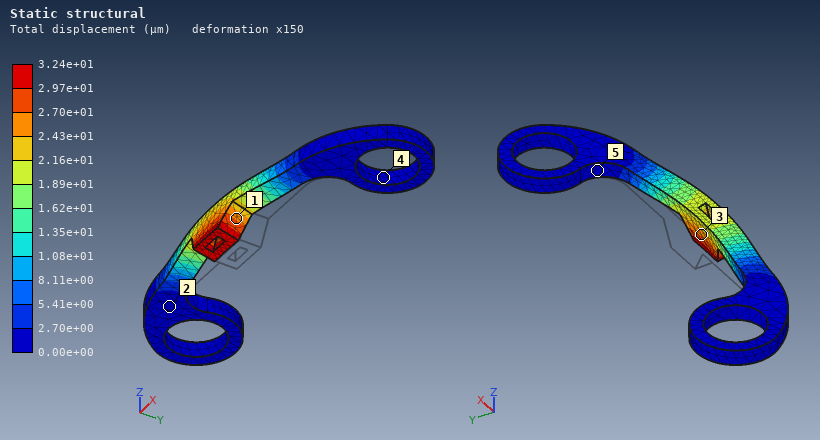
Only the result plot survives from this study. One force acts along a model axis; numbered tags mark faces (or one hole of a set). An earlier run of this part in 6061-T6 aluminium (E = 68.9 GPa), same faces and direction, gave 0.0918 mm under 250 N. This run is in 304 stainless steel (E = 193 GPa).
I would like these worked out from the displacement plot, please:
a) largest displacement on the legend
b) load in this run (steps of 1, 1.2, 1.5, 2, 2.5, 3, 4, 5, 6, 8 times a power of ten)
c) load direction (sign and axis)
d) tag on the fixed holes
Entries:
3.24e+01 µm
250 N
-Y
4
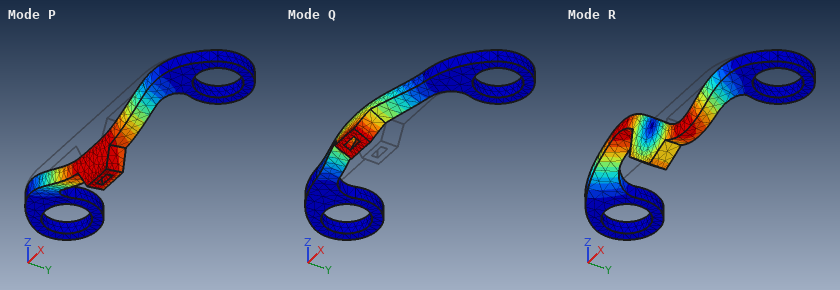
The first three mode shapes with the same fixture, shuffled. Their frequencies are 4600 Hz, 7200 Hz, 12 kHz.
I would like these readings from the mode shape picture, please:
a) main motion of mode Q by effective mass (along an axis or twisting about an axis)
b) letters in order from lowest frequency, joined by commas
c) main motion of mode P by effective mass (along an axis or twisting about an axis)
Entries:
along Y
P, Q, R
along Z
